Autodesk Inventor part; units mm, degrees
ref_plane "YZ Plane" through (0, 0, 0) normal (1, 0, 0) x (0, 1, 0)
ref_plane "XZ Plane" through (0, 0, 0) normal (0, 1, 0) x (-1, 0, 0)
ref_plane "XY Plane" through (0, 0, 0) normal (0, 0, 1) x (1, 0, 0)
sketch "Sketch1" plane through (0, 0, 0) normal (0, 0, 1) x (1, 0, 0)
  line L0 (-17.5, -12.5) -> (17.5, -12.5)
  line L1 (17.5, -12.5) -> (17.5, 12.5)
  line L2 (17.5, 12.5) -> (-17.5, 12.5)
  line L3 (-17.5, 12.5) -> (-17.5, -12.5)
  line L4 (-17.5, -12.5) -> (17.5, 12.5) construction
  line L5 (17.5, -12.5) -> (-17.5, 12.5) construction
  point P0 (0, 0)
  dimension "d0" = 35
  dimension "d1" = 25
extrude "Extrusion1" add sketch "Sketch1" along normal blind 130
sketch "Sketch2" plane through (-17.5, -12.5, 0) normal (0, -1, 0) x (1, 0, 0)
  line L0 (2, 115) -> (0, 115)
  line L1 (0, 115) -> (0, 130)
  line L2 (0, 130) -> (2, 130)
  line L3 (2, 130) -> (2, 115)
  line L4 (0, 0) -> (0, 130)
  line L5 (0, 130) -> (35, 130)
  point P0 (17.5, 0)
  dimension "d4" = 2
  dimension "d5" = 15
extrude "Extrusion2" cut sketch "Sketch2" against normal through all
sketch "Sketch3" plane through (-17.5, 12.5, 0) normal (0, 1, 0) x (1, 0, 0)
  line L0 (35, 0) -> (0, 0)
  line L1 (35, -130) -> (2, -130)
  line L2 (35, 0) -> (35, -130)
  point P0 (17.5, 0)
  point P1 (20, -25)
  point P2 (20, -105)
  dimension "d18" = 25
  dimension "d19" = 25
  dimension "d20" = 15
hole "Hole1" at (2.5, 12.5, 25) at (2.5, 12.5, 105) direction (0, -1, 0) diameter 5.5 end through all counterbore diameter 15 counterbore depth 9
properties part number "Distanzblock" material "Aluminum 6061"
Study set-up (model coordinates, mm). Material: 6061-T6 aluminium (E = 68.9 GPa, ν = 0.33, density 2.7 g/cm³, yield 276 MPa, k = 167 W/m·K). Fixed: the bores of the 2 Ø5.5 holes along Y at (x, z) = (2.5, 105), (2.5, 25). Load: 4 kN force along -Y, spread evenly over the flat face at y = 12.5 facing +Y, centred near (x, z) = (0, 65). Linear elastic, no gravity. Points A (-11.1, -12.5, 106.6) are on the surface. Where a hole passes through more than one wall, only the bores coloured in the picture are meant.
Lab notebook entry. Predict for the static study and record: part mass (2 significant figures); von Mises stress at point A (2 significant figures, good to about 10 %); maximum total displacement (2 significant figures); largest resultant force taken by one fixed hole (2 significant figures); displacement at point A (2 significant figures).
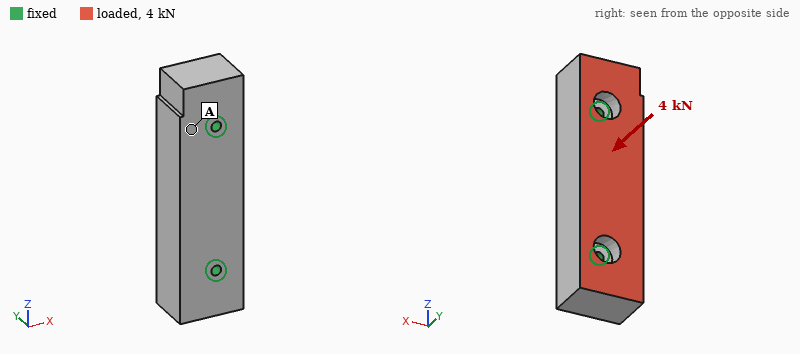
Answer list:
290 g
2.6 MPa
5.6 µm
2.0 kN
2.1 µm
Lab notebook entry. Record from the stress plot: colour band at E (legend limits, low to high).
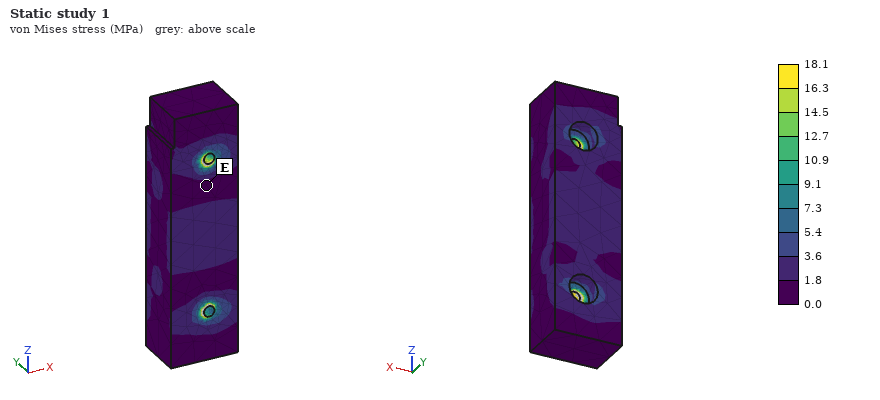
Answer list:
0.0 to 1.8 MPa
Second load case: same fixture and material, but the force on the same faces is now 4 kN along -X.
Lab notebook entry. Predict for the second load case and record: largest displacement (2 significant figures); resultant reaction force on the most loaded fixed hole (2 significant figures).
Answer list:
15 µm
2.0 kN
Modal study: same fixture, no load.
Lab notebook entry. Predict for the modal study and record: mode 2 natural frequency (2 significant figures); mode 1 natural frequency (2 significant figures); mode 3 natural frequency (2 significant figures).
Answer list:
9500 Hz
8300 Hz
9900 Hz
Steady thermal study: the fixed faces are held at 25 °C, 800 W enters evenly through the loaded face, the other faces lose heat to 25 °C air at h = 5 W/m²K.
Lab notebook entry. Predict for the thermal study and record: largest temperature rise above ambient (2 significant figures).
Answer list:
75 K
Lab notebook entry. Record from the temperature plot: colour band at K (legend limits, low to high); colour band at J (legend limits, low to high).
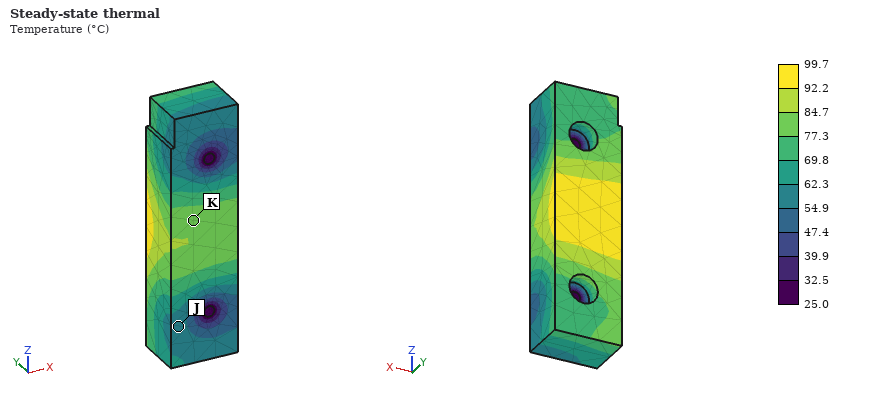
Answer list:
77.3 to 84.7 °C
54.9 to 62.3 °C
